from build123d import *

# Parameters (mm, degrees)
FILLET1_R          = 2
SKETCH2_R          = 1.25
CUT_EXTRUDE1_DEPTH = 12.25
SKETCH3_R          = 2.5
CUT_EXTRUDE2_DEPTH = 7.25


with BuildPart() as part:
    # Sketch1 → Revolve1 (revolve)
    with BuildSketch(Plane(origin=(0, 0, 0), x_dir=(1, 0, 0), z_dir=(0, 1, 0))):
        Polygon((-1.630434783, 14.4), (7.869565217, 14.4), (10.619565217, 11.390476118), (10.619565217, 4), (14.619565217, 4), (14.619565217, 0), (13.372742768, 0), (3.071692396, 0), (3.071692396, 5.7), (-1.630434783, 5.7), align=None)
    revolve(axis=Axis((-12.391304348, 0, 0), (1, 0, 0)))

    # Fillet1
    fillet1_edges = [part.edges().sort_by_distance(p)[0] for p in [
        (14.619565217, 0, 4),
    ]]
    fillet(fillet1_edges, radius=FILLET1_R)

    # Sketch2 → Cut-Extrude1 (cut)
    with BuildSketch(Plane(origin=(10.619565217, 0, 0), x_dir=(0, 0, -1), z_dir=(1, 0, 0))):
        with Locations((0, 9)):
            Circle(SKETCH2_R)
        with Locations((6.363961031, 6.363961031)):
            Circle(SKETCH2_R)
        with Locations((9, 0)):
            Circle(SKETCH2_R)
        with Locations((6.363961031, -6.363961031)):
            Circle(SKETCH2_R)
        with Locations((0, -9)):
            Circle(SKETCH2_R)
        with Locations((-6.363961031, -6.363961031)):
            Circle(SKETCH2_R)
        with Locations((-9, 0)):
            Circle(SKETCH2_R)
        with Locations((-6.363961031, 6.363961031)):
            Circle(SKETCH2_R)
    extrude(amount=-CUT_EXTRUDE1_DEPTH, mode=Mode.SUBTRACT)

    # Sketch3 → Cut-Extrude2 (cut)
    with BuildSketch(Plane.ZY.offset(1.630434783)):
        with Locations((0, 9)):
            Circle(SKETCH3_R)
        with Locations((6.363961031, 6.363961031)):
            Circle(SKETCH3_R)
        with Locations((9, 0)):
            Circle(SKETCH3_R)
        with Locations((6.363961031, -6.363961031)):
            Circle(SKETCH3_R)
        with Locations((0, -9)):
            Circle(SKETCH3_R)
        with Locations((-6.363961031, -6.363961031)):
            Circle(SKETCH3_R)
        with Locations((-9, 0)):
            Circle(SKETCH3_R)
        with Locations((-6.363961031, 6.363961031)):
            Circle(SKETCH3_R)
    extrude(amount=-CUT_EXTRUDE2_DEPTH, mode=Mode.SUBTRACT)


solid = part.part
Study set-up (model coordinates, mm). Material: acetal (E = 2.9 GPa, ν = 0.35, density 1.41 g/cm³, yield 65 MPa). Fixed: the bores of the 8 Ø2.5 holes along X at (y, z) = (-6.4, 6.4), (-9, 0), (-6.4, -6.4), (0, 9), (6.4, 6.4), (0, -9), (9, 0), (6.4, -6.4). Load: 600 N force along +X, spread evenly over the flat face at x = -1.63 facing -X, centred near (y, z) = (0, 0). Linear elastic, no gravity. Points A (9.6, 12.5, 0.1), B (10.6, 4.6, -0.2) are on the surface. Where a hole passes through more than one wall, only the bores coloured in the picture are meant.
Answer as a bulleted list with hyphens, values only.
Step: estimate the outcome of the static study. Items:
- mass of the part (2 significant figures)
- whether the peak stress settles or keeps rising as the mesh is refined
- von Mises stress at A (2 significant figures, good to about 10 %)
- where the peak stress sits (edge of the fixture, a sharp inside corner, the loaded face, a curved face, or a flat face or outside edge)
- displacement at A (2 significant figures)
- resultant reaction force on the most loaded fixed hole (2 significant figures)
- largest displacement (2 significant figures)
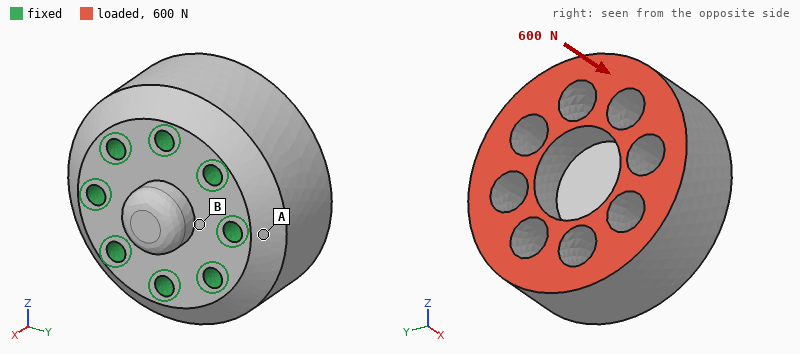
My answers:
- 8.5 g
- keeps rising
- 1.5 MPa
- edge of the fixture
- 4.0 µm
- 75 N
- 12 µm
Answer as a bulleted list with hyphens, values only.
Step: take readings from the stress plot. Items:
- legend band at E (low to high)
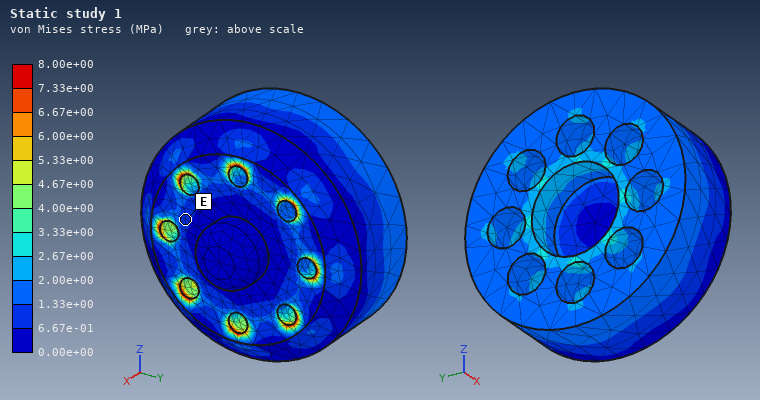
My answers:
- 6.67e-01 to 1.33e+00 MPa
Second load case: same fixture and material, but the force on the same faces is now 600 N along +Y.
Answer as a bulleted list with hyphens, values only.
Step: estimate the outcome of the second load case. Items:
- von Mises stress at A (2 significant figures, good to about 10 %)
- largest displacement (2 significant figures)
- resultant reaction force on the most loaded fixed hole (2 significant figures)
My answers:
- 4.5 MPa
- 50 µm
- 130 N
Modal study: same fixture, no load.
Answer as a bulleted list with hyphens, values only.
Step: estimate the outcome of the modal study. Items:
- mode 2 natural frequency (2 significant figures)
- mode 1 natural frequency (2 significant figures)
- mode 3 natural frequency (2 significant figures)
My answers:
- 14 kHz
- 14 kHz
- 15 kHz
